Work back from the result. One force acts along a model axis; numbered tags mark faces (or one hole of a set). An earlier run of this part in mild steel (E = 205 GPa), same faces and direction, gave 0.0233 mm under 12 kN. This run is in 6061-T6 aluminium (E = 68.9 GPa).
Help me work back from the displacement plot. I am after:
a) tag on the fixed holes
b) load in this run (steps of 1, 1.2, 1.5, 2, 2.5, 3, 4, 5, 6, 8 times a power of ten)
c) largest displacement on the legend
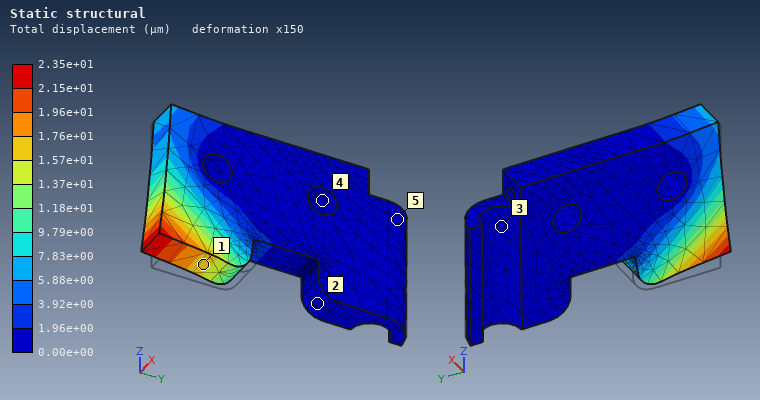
4
4 kN
2.35e+01 µm
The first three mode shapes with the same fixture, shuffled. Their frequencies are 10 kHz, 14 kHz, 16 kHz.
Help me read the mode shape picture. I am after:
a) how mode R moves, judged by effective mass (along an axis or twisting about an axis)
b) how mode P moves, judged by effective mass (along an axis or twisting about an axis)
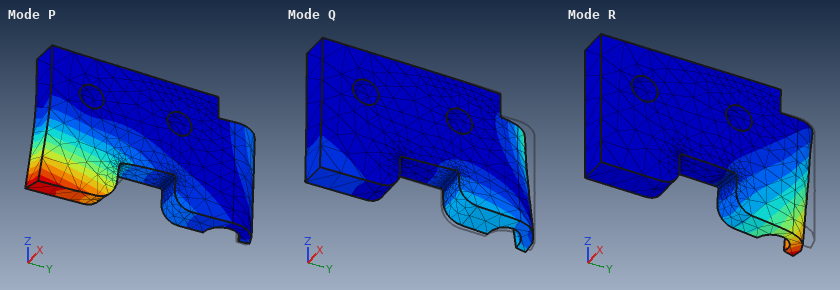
along X
along X
